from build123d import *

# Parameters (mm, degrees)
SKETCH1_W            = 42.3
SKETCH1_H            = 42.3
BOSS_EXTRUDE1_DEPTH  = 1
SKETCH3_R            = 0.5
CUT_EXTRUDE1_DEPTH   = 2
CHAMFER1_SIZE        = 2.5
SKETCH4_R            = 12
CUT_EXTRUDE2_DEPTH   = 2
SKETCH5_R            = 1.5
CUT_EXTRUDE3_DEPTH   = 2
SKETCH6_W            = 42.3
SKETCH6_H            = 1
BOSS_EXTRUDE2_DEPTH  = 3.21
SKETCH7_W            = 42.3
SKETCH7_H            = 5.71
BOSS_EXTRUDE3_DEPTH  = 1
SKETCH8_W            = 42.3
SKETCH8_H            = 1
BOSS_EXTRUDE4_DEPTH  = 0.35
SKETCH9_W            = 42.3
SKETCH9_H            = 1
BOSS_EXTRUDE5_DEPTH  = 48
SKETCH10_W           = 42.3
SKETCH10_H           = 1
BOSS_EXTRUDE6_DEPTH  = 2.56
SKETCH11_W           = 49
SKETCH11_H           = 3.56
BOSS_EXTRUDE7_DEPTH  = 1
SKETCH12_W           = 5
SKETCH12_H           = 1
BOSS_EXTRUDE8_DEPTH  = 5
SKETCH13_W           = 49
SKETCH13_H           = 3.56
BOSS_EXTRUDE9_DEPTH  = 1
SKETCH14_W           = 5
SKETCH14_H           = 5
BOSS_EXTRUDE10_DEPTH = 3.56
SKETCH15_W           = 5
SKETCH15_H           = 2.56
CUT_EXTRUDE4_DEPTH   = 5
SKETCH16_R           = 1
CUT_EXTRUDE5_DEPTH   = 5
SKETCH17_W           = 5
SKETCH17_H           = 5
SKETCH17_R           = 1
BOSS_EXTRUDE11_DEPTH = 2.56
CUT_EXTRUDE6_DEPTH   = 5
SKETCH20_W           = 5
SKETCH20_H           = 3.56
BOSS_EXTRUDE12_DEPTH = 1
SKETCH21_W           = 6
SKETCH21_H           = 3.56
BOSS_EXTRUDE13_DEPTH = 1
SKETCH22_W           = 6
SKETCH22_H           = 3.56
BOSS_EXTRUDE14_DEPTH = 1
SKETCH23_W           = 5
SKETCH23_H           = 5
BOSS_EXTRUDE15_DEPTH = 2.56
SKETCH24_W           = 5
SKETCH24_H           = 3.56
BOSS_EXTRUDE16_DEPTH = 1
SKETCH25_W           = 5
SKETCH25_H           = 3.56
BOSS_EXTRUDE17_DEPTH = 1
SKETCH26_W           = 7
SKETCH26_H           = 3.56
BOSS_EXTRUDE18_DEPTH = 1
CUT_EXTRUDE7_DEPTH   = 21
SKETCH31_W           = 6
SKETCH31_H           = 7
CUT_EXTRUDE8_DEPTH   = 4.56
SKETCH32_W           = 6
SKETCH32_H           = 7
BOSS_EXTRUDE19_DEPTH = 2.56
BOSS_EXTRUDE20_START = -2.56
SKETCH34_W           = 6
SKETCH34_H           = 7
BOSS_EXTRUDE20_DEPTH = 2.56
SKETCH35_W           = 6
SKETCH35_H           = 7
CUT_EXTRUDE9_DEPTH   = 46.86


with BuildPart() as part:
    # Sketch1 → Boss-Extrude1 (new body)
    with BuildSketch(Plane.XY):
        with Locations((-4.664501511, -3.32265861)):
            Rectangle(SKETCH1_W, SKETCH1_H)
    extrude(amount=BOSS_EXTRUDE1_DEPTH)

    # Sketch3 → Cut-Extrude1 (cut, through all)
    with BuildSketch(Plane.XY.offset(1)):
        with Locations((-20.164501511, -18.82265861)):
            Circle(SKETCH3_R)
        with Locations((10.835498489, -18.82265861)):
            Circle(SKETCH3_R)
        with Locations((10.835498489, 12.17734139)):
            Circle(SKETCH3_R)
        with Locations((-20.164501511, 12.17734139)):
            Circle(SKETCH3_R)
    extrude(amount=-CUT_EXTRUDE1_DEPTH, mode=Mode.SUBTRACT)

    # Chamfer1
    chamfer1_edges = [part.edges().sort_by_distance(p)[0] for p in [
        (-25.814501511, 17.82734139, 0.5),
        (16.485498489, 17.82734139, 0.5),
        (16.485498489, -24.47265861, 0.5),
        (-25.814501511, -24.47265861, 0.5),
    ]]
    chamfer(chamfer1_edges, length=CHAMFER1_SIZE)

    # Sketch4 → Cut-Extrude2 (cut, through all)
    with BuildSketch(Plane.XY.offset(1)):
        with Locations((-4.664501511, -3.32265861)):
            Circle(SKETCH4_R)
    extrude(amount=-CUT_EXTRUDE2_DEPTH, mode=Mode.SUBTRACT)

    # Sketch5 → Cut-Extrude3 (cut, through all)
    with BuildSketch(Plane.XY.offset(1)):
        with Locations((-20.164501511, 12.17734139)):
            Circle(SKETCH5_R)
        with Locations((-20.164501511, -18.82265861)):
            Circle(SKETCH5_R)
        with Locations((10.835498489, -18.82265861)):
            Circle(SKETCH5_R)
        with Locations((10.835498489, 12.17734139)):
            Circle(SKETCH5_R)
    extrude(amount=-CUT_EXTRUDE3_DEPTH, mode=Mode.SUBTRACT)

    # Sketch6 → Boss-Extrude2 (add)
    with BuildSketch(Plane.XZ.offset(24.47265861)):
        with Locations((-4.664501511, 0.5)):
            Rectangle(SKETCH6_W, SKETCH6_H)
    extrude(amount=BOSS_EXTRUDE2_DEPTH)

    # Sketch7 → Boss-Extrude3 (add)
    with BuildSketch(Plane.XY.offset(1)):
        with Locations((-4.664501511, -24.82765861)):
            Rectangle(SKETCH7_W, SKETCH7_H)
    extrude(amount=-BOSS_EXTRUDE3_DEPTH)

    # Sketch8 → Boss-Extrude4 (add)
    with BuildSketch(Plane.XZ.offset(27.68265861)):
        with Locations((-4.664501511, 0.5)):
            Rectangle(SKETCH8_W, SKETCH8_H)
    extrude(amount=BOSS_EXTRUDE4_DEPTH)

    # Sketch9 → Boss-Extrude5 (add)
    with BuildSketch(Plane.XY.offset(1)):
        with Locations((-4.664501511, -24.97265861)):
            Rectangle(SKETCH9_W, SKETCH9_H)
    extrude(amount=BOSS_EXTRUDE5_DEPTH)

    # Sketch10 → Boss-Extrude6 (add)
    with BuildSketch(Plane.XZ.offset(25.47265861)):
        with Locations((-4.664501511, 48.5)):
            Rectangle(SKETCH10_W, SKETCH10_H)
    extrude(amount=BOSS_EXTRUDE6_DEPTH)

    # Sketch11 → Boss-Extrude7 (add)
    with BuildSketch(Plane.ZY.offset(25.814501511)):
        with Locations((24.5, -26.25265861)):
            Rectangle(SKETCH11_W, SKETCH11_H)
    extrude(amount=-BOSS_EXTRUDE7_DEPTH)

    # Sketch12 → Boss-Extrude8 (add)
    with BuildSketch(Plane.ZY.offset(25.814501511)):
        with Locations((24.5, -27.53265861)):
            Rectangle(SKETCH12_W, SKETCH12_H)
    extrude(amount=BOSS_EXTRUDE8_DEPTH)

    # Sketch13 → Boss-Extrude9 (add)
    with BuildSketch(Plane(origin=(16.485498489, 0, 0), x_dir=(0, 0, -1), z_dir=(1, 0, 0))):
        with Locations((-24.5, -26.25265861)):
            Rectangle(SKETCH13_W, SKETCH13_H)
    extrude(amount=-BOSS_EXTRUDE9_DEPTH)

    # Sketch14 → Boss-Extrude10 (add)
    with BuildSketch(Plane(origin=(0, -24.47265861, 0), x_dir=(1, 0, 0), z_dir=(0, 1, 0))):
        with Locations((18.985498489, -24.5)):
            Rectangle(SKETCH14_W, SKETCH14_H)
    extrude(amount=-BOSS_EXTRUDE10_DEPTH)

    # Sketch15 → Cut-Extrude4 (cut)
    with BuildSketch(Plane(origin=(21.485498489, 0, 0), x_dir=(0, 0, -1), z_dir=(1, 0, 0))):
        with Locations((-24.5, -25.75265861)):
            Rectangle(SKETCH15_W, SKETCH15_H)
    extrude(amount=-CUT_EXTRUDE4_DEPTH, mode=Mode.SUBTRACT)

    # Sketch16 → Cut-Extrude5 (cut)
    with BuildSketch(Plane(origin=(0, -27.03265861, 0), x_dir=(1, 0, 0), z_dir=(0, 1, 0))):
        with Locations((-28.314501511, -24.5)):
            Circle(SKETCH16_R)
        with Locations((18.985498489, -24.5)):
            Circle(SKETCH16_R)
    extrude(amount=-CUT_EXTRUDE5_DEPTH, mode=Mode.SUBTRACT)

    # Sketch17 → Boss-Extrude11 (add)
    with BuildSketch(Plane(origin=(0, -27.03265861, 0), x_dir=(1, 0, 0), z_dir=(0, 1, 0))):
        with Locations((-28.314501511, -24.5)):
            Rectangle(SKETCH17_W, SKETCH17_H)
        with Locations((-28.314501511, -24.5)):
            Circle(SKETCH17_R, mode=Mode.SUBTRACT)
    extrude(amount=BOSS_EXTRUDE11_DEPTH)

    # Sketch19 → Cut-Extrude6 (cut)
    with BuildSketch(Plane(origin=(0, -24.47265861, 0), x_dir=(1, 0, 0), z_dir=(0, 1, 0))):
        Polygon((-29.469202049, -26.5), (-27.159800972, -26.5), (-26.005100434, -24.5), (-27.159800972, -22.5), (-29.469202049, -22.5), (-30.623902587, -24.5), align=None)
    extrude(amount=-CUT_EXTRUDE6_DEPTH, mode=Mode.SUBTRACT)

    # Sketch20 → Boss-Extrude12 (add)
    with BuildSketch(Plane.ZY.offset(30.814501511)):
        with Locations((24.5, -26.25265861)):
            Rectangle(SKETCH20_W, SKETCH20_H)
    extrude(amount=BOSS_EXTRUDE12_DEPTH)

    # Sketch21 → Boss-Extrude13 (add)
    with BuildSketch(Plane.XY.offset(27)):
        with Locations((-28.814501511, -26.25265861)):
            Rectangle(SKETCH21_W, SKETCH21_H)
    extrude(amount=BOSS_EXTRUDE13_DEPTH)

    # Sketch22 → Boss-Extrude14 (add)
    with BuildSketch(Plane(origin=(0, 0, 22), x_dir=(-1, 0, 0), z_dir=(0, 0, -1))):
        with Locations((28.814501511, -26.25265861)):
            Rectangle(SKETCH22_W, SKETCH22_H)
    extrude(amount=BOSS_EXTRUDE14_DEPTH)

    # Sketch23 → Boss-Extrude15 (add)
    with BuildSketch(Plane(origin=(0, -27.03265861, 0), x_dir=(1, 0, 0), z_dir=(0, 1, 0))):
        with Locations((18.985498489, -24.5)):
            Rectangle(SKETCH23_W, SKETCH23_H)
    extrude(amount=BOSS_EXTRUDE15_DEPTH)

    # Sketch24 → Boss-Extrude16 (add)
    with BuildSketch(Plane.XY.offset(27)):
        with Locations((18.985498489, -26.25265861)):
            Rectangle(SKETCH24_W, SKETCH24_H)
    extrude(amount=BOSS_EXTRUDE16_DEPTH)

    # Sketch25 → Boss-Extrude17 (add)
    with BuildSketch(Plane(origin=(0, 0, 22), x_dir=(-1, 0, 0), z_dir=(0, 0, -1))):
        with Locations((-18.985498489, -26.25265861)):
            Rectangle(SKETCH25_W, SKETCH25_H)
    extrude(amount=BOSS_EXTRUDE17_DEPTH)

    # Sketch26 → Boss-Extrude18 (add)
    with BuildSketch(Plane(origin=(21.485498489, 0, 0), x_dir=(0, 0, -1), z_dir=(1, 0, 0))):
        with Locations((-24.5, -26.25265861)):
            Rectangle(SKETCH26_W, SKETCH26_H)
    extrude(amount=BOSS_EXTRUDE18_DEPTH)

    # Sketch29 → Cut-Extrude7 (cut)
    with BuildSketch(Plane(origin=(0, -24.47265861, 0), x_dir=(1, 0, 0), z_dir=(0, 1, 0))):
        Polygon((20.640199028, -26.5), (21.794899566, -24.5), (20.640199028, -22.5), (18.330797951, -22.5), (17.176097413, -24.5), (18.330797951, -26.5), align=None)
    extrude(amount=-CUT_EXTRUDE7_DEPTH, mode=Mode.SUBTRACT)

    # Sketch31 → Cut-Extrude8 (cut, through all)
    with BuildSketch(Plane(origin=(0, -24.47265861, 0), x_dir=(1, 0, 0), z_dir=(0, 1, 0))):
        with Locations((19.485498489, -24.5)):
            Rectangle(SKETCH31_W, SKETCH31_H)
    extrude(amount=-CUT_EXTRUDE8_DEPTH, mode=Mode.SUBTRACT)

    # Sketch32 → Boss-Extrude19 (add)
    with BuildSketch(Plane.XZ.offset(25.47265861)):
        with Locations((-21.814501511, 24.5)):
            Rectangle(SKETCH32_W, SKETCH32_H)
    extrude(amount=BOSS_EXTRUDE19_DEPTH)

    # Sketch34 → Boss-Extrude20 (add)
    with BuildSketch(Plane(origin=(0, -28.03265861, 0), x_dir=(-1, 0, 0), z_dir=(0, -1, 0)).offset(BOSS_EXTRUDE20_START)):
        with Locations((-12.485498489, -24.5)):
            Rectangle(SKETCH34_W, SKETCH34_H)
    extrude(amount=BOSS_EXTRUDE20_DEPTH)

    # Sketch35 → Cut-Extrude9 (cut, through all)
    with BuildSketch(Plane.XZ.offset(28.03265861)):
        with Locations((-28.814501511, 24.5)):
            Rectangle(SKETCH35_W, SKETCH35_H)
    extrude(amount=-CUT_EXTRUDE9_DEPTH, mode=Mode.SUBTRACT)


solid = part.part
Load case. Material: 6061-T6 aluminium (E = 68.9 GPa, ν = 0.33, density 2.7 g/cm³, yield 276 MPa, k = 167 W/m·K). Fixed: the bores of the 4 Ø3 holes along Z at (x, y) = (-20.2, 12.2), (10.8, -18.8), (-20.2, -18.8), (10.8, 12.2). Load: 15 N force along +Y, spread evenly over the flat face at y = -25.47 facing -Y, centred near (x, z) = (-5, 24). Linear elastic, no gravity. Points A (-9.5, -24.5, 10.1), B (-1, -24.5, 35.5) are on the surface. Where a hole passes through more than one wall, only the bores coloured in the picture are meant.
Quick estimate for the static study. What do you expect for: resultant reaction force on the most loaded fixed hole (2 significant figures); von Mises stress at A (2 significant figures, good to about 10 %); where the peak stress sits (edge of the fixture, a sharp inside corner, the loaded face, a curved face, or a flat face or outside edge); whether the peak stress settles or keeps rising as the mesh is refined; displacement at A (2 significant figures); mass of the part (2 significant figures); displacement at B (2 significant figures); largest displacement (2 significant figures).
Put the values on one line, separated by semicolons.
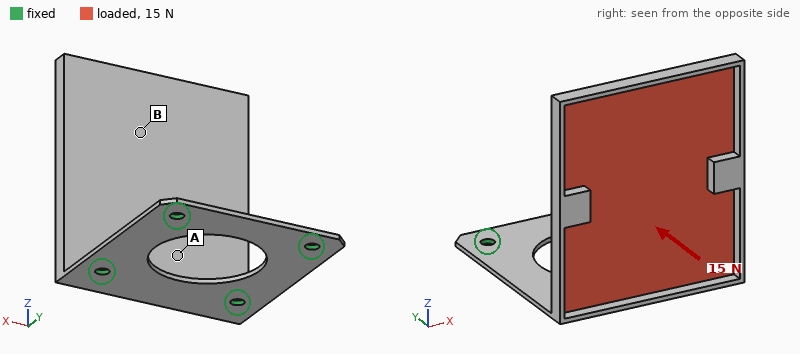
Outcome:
11 N; 12 MPa; edge of the fixture; keeps rising; 0.11 mm; 11 g; 0.50 mm; 0.71 mm
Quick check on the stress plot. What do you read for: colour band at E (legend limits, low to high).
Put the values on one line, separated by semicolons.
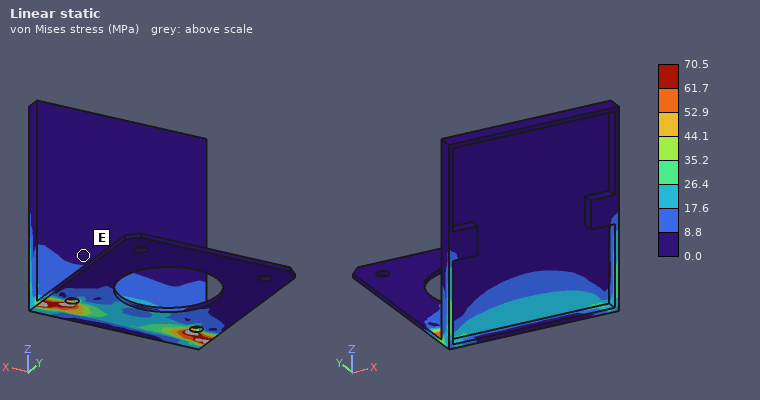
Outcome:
0.0 to 8.8 MPa
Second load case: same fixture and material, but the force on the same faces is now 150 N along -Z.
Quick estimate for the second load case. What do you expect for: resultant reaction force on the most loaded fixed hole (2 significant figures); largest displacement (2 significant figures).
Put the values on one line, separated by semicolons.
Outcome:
76 N; 0.74 mm
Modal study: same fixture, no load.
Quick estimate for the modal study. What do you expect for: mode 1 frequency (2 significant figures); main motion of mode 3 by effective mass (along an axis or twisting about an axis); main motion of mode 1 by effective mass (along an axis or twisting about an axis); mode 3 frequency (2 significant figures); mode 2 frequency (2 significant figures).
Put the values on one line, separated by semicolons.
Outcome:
330 Hz; along X; along Y; 2100 Hz; 880 Hz
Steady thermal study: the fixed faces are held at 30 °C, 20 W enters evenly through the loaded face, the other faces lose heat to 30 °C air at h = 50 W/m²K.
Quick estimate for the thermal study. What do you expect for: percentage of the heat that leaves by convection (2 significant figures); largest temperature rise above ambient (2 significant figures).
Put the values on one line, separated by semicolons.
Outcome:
37 %; 52 K
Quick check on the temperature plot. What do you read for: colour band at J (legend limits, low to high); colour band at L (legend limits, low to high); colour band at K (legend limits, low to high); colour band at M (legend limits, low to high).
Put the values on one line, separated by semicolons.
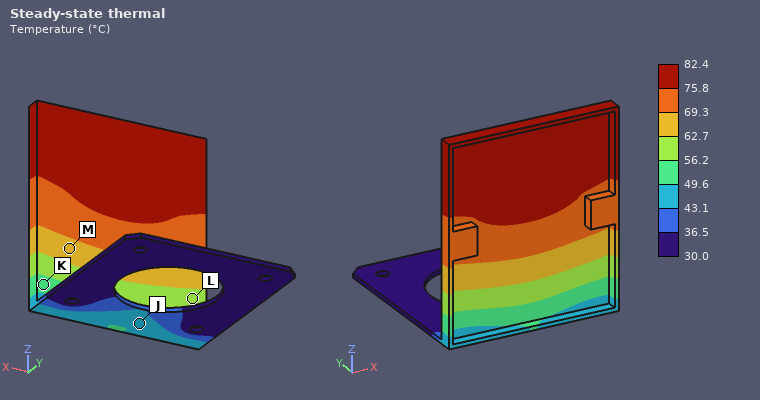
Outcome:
43.1 to 49.6 °C; 56.2 to 62.7 °C; 49.6 to 56.2 °C; 62.7 to 69.3 °C
